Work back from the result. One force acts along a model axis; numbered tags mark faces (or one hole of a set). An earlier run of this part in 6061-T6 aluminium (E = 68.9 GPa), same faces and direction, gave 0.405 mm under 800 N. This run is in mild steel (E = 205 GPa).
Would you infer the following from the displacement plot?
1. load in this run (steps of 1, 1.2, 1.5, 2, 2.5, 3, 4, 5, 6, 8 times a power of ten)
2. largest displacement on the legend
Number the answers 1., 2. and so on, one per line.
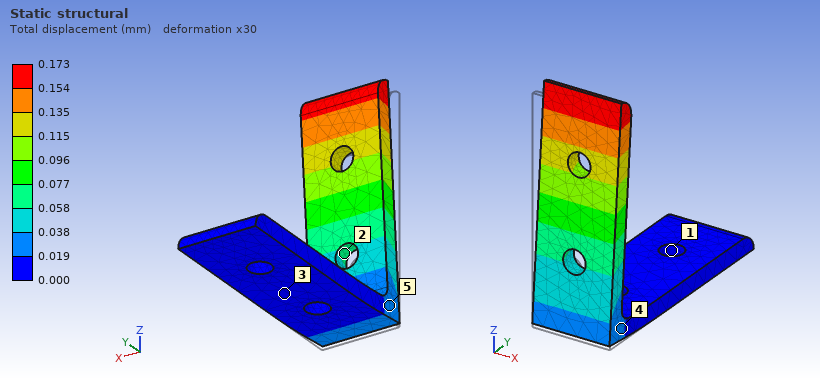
1. 1 kN
2. 0.173 mm
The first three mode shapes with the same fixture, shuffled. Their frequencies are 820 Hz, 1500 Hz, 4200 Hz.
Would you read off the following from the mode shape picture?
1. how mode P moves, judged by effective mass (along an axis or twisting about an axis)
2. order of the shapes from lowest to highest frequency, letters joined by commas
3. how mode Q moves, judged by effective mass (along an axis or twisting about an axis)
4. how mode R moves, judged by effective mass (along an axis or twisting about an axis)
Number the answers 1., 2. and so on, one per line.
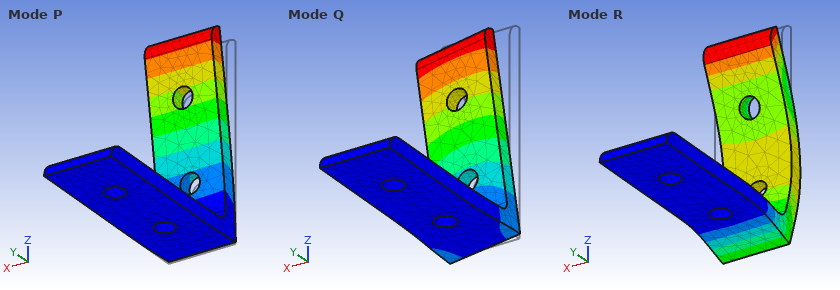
1. along Y
2. P, Q, R
3. along X
4. along Z
